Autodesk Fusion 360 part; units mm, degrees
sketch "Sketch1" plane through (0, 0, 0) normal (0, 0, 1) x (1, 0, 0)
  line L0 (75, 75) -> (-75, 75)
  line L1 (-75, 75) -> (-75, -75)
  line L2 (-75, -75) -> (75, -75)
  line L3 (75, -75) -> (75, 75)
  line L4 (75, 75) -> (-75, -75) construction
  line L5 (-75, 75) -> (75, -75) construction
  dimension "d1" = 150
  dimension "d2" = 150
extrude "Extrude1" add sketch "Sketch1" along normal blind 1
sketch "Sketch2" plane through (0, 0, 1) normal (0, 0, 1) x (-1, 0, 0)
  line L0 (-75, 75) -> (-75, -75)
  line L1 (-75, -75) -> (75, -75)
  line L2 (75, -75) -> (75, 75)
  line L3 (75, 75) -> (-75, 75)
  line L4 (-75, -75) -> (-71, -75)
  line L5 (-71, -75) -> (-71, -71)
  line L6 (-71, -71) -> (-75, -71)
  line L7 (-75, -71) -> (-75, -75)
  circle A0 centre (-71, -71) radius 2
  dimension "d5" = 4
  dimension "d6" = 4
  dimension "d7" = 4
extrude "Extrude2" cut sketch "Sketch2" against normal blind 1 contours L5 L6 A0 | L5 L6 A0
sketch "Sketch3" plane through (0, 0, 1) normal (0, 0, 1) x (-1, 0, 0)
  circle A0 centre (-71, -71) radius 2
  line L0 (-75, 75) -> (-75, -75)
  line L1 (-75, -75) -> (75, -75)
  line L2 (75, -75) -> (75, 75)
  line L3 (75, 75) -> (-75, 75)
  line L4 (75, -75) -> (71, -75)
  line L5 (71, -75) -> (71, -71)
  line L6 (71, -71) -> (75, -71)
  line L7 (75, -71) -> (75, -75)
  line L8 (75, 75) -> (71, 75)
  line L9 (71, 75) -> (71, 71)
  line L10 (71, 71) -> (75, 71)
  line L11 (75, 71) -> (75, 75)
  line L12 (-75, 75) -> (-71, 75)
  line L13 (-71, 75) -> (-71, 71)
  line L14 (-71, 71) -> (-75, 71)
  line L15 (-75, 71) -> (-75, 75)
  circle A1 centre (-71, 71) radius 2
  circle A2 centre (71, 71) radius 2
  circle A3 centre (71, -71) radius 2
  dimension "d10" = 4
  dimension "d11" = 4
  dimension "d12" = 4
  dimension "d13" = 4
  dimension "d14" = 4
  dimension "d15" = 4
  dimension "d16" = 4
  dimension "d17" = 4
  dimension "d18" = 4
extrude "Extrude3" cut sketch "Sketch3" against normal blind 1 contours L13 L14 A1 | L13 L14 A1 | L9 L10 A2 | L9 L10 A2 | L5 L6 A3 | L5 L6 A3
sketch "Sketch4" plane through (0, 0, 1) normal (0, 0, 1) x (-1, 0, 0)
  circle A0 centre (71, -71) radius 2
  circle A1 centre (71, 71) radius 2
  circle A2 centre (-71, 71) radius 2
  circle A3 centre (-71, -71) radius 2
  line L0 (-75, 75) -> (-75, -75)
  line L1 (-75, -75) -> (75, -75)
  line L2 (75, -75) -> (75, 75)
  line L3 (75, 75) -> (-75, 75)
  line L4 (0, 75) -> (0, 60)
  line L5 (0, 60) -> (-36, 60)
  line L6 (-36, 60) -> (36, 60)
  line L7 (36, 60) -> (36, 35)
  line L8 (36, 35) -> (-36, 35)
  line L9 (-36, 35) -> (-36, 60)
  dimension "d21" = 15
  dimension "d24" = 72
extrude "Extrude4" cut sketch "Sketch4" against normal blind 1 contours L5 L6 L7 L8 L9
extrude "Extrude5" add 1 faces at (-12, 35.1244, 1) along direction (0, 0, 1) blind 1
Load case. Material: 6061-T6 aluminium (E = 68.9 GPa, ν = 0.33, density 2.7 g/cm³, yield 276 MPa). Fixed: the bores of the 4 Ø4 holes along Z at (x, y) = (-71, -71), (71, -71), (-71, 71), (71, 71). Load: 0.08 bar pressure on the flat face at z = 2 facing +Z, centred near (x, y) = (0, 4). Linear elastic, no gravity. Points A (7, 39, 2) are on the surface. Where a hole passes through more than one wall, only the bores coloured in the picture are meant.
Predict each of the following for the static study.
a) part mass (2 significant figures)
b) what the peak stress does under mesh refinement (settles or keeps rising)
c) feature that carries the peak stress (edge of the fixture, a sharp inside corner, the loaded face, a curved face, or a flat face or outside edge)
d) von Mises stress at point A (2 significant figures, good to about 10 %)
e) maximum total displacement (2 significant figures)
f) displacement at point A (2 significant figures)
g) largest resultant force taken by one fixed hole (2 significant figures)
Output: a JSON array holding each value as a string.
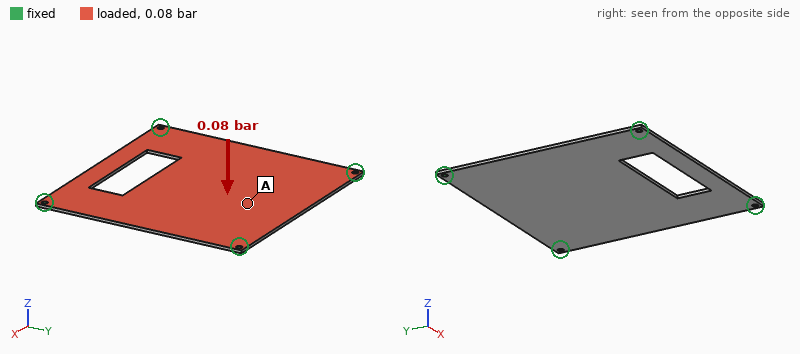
["110 g", "keeps rising", "edge of the fixture", "14 MPa", "0.63 mm", "0.50 mm", "44 N"]
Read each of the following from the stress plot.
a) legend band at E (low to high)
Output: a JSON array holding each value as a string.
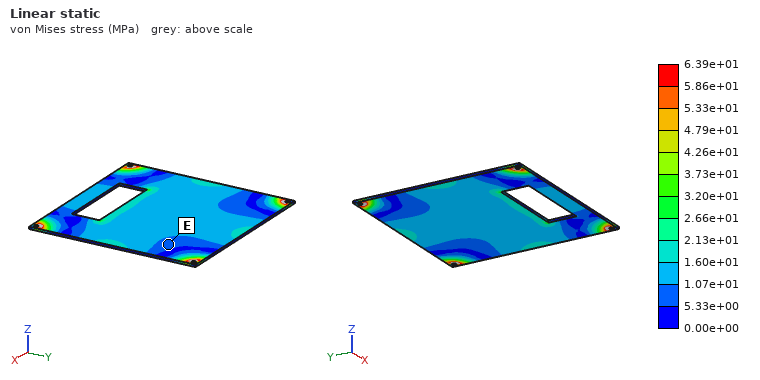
["5.33e+00 to 1.07e+01 MPa"]
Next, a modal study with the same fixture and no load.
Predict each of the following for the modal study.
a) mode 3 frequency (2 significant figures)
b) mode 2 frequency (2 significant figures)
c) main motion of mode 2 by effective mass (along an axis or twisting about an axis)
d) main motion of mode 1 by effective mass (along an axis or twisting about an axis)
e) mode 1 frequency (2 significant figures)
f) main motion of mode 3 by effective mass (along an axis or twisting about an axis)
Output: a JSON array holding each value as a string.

["570 Hz", "530 Hz", "twisting about Y", "along Z", "290 Hz", "twisting about X"]
